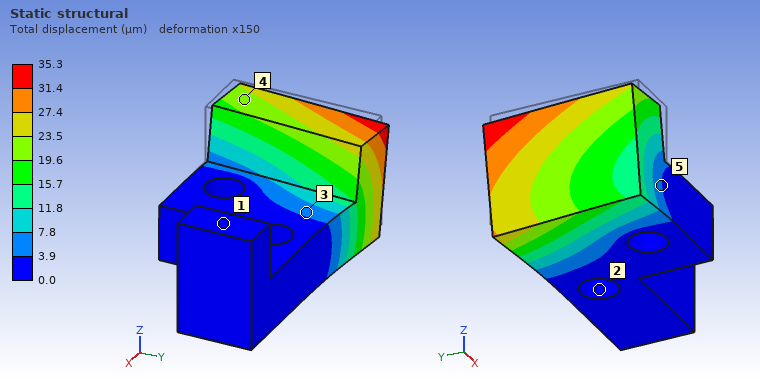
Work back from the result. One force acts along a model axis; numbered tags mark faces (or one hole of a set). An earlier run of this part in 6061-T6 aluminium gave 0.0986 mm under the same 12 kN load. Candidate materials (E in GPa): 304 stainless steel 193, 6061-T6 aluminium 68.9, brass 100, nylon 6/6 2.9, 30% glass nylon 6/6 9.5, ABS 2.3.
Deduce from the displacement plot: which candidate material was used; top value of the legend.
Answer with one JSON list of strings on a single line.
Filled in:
["304 stainless steel", "35.3 µm"]
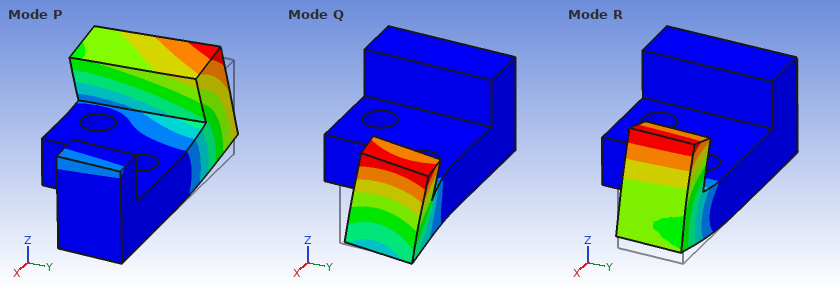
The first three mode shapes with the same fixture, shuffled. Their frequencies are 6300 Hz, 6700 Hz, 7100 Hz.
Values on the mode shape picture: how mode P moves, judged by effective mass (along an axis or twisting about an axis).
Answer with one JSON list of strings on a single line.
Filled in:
["along Z"]
